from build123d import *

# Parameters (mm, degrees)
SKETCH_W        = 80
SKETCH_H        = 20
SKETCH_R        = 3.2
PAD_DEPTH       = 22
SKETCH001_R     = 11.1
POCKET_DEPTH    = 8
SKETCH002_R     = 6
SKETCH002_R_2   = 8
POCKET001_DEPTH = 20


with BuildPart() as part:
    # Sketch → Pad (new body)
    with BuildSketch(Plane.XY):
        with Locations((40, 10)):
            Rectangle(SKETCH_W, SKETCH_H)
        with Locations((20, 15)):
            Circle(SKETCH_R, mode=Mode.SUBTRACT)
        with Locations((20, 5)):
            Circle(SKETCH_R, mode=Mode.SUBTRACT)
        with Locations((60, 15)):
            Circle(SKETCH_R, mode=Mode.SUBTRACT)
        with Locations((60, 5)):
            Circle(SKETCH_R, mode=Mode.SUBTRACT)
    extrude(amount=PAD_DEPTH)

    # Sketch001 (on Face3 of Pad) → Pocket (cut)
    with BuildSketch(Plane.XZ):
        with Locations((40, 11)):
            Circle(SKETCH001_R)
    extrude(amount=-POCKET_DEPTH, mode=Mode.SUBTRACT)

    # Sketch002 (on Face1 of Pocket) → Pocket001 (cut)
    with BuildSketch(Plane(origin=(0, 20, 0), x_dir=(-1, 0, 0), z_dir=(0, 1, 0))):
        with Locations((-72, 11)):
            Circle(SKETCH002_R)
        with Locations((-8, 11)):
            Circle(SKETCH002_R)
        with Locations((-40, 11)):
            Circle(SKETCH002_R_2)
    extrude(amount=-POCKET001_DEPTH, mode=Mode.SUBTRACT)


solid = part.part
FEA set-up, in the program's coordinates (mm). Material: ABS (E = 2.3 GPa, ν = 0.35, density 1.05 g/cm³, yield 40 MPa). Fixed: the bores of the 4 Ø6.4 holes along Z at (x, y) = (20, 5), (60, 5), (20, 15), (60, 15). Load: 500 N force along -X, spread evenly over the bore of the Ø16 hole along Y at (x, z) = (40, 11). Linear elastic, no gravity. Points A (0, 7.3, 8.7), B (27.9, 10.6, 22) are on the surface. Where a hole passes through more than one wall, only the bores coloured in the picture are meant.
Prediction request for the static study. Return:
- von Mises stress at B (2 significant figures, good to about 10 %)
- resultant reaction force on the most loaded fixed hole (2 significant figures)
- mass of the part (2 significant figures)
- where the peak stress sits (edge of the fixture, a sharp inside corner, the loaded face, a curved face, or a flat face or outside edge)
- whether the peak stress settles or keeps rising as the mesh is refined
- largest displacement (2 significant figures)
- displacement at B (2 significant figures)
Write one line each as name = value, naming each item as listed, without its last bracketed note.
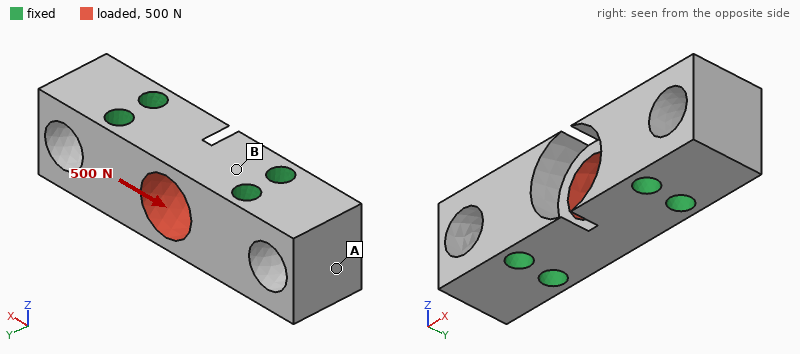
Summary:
von Mises stress at B = 0.80 MPa
resultant reaction force on the most loaded fixed hole = 190 N
mass of the part = 23 g
where the peak stress sits = edge of the fixture
whether the peak stress settles or keeps rising as the mesh is refined = keeps rising
largest displacement = 7.2 µm
displacement at B = 2.4 µm
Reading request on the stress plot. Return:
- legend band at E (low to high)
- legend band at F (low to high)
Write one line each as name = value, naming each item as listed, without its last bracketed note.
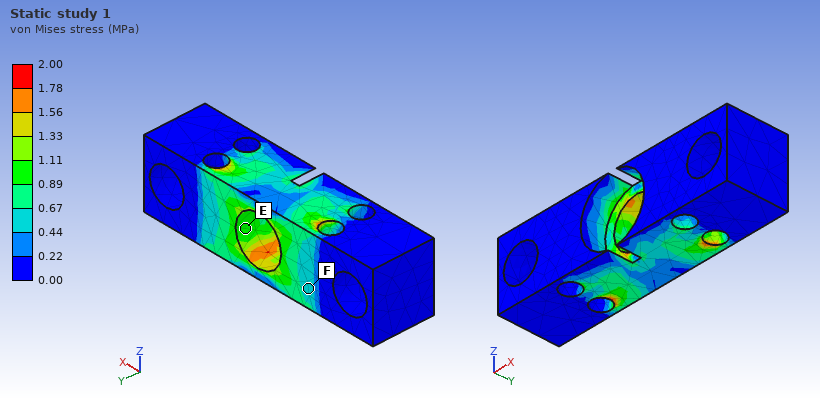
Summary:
legend band at E = 0.89 to 1.11 MPa
legend band at F = 0.44 to 0.67 MPa
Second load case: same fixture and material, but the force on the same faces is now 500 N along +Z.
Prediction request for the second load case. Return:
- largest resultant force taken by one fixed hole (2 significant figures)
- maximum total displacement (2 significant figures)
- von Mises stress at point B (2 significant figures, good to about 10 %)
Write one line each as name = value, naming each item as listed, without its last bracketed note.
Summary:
largest resultant force taken by one fixed hole = 170 N
maximum total displacement = 34 µm
von Mises stress at point B = 1.3 MPa
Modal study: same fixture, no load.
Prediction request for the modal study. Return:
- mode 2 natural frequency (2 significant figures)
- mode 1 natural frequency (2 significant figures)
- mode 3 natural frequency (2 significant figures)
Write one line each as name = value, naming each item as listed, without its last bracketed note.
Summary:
mode 2 natural frequency = 6200 Hz
mode 1 natural frequency = 6200 Hz
mode 3 natural frequency = 8000 Hz
